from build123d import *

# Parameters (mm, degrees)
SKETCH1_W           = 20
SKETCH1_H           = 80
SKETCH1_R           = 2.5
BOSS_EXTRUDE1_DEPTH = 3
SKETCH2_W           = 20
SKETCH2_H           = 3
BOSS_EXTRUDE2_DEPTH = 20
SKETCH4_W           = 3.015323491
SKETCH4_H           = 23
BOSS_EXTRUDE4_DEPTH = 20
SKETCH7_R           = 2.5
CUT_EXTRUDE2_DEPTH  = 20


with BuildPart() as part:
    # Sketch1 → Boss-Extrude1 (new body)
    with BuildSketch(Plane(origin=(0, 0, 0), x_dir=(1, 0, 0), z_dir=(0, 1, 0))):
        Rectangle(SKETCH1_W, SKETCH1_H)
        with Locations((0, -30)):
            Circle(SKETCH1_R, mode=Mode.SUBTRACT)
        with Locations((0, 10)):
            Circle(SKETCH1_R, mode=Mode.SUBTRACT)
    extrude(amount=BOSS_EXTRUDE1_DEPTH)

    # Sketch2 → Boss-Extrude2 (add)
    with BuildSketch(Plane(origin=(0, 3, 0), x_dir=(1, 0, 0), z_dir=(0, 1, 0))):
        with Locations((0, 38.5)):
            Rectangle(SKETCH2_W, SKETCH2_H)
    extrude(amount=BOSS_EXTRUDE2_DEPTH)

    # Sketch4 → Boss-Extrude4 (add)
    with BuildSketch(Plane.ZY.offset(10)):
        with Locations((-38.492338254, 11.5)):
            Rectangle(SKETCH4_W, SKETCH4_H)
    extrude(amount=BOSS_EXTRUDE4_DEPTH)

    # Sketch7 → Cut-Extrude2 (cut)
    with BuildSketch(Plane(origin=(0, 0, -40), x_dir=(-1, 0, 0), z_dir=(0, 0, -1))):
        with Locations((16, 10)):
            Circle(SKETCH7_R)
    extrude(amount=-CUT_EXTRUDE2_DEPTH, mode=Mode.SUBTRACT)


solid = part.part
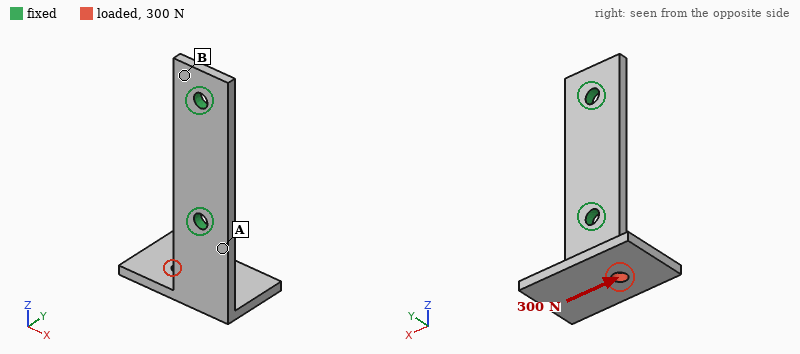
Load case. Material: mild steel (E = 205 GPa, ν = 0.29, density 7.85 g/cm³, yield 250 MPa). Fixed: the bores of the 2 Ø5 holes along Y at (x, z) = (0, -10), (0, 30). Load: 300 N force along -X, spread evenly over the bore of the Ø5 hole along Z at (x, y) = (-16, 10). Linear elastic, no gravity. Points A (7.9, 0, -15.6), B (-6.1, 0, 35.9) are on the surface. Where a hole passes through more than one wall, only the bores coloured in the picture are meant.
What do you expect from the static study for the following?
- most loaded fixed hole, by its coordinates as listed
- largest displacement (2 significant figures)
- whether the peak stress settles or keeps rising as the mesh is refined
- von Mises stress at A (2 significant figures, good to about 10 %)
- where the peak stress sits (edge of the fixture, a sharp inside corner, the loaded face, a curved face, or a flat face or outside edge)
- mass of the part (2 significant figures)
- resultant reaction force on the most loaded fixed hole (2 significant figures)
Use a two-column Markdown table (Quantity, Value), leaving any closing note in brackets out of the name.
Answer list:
| Quantity | Value |
|---|---|
| most loaded fixed hole, by its coordinates as listed | (0, -10) |
| largest displacement | 0.18 mm |
| whether the peak stress settles or keeps rising as the mesh is refined | keeps rising |
| von Mises stress at A | 65 MPa |
| where the peak stress sits | edge of the fixture |
| mass of the part | 57 g |
| resultant reaction force on the most loaded fixed hole | 430 N |
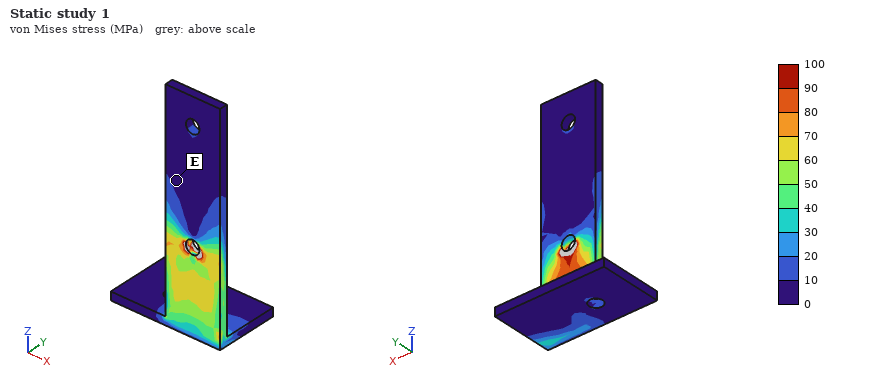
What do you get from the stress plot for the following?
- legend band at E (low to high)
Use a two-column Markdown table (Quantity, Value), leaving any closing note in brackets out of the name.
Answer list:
| Quantity | Value |
|---|---|
| legend band at E | 0 to 10 MPa |
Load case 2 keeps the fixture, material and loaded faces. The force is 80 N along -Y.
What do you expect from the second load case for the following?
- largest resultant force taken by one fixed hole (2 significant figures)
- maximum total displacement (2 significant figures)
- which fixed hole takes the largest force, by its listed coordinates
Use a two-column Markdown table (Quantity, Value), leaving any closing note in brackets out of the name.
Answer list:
| Quantity | Value |
|---|---|
| largest resultant force taken by one fixed hole | 83 N |
| maximum total displacement | 0.16 mm |
| which fixed hole takes the largest force, by its listed coordinates | (0, -10) |
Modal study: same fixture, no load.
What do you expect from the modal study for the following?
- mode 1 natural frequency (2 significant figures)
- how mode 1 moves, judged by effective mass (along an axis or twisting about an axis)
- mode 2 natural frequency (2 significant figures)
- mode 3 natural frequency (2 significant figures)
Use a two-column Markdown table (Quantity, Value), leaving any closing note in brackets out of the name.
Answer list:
| Quantity | Value |
|---|---|
| mode 1 natural frequency | 920 Hz |
| how mode 1 moves, judged by effective mass | along Y |
| mode 2 natural frequency | 1500 Hz |
| mode 3 natural frequency | 2700 Hz |
